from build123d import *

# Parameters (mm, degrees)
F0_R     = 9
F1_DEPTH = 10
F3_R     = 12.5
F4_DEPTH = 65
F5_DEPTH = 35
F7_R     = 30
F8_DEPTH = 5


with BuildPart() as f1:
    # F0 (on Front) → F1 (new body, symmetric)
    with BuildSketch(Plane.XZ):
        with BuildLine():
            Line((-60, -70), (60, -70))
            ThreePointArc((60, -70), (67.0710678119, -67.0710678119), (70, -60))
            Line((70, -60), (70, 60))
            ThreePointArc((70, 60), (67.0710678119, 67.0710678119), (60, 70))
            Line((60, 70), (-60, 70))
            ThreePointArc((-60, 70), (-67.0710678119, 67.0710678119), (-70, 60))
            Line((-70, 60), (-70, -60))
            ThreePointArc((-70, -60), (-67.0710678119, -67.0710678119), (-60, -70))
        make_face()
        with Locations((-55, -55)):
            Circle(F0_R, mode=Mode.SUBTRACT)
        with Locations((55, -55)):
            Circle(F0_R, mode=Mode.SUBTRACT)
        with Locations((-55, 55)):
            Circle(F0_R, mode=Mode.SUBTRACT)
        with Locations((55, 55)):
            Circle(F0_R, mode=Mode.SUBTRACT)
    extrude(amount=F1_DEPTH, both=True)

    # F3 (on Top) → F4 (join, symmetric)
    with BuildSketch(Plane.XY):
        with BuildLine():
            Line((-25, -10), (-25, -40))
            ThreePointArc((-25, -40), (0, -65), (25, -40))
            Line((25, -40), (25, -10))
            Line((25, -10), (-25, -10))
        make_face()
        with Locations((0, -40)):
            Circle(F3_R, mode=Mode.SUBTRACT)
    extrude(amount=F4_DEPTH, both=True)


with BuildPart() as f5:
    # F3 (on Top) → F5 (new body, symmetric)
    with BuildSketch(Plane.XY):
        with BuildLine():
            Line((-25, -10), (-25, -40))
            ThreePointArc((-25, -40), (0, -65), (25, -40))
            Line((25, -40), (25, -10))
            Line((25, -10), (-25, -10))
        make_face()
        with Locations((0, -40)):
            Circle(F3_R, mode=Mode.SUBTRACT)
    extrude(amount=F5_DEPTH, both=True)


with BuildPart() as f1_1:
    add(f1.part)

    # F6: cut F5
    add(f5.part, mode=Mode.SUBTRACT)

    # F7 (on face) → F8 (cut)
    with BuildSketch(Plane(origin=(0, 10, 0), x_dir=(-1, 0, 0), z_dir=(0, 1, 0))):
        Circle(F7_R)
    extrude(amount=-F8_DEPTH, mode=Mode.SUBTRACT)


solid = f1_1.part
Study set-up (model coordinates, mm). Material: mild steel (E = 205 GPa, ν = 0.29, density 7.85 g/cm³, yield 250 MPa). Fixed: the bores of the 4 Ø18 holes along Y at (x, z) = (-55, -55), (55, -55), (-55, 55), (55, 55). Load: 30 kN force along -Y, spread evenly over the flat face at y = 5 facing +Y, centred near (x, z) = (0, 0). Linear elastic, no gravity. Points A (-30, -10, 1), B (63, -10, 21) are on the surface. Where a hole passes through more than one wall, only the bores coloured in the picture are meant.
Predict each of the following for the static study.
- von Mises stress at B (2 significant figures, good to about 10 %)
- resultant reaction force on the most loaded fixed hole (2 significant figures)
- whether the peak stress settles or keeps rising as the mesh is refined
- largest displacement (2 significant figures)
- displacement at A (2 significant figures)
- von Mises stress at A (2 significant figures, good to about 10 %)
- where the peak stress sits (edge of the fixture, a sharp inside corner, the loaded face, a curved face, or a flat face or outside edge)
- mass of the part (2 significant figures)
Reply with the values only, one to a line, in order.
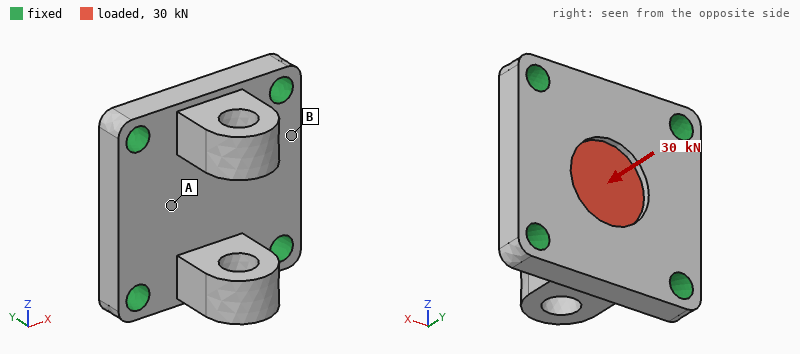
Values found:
13 MPa
8.0 kN
keeps rising
35 µm
24 µm
39 MPa
edge of the fixture
3.7 kg
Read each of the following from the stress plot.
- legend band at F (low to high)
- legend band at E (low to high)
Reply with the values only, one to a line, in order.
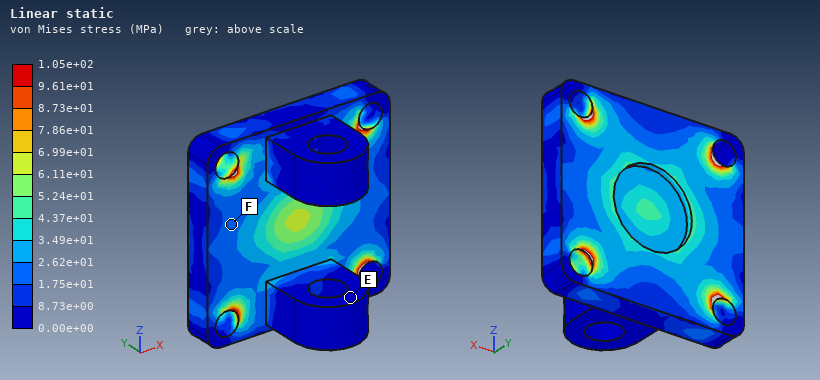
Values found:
1.75e+01 to 2.62e+01 MPa
0.00e+00 to 8.73e+00 MPa
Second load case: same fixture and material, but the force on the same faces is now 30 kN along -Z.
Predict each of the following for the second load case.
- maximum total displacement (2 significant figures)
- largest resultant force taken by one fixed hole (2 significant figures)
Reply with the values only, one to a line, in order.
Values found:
5.7 µm
8.3 kN
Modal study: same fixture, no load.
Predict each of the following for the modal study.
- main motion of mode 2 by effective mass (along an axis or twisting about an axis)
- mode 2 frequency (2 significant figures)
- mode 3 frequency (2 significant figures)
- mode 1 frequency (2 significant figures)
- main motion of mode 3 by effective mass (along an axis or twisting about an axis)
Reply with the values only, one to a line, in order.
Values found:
along Z
4500 Hz
6100 Hz
3800 Hz
along Y
